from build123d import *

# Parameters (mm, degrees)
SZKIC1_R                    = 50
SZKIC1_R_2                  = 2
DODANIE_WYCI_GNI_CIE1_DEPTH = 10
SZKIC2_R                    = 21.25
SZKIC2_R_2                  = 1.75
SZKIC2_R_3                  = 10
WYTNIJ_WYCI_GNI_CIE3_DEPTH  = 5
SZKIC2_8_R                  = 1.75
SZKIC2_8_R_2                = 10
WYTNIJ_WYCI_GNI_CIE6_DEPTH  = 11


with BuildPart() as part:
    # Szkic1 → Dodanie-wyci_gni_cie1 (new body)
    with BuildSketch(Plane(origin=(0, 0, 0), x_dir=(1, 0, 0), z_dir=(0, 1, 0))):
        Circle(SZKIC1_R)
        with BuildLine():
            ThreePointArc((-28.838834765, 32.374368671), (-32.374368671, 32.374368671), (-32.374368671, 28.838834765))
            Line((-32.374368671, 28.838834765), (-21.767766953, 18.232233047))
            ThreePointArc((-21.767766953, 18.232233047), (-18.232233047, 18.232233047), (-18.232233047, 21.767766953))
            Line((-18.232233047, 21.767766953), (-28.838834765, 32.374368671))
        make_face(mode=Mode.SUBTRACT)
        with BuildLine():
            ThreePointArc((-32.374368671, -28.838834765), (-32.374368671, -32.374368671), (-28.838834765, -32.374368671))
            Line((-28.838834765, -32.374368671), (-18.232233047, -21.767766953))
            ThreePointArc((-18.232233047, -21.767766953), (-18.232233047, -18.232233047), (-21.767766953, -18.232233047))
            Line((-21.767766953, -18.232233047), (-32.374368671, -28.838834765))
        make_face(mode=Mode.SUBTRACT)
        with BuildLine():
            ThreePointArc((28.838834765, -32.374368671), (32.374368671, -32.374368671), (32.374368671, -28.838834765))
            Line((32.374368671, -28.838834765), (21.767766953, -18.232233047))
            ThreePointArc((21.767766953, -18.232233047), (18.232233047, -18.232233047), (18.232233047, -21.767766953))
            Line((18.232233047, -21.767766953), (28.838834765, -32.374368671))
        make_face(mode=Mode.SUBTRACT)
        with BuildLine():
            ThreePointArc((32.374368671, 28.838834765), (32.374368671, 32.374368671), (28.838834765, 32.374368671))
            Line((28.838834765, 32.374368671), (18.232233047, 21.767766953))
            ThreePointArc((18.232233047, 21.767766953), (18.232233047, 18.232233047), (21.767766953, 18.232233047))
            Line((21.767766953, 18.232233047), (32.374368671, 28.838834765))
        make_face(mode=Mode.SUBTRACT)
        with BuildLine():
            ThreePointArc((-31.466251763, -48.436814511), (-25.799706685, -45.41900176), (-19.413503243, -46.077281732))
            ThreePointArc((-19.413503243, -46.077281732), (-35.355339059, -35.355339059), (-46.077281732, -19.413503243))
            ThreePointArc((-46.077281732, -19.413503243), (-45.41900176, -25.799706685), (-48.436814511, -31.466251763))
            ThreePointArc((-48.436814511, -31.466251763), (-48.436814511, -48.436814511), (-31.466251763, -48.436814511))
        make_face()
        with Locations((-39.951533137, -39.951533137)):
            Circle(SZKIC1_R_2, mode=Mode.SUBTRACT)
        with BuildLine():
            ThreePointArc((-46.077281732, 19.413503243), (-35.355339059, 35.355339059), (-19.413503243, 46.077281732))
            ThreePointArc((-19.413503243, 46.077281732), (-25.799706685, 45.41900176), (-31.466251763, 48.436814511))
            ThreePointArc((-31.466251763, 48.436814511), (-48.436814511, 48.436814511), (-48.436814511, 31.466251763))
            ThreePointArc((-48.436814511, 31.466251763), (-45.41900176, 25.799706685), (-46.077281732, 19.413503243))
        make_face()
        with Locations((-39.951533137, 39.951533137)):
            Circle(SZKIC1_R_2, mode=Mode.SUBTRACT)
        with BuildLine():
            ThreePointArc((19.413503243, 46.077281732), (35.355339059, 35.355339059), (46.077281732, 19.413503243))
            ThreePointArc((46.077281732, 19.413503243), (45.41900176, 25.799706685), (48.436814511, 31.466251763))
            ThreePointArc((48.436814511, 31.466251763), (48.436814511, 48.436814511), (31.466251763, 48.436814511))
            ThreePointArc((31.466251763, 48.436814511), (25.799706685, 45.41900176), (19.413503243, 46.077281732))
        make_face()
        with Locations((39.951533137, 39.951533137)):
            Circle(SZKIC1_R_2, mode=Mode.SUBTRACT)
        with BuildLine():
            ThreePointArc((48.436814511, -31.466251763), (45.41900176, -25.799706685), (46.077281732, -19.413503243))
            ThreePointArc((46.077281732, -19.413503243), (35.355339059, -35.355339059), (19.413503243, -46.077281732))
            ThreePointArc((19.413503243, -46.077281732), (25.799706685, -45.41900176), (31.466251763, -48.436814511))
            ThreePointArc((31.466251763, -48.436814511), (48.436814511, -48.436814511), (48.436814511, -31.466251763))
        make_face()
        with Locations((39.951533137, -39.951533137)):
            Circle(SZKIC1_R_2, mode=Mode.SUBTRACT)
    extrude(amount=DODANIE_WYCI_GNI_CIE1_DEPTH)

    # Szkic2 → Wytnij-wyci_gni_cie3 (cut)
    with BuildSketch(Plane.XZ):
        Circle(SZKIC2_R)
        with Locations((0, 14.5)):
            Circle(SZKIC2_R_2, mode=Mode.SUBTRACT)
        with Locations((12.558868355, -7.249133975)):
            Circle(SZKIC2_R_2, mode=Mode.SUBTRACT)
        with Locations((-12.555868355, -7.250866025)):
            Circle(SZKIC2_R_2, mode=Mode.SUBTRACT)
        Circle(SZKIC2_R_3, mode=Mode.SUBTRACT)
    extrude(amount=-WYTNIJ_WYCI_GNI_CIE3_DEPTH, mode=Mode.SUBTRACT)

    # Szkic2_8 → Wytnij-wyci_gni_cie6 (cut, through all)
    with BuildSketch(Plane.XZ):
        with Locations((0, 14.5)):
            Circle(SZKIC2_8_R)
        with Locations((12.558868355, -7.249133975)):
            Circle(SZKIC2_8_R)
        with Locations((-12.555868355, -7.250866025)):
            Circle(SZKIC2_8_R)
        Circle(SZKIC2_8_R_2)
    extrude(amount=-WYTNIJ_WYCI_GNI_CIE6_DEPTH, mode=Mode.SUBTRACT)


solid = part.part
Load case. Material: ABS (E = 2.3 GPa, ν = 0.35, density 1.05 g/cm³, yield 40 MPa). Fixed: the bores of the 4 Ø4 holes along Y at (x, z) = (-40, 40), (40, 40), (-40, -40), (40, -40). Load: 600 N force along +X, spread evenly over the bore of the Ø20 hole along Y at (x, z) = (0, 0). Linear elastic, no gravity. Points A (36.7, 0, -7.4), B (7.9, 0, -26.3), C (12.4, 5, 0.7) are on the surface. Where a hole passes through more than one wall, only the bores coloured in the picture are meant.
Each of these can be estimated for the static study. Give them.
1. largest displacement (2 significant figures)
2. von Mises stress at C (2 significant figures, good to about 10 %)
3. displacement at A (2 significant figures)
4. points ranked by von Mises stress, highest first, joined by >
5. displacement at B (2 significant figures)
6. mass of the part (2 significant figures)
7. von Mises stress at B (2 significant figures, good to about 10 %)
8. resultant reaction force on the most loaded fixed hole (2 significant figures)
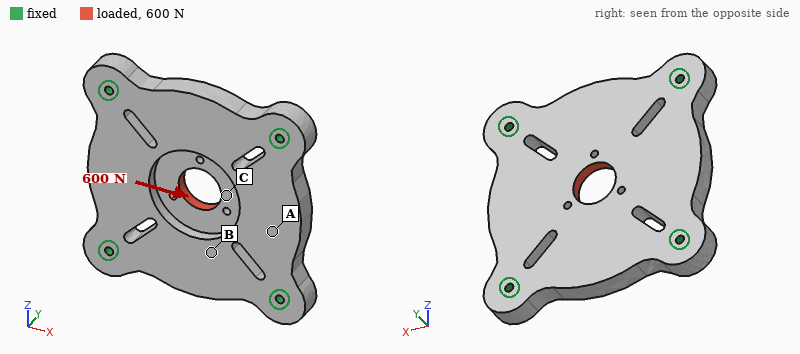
37 µm
1.8 MPa
20 µm
C > B > A
12 µm
86 g
0.79 MPa
170 N
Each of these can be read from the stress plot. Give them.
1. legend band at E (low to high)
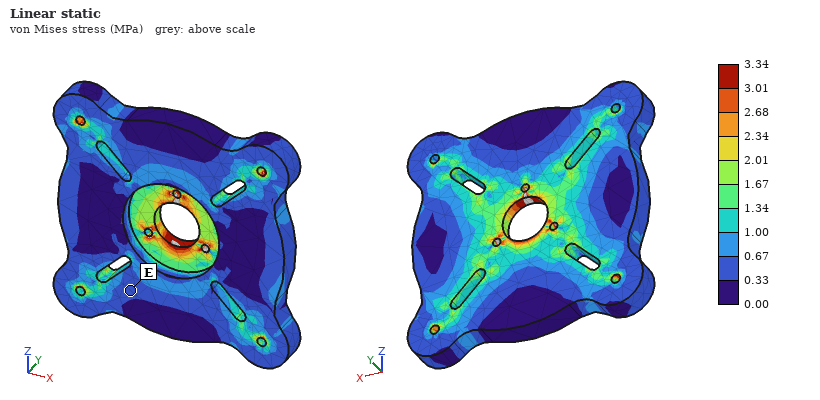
0.33 to 0.67 MPa
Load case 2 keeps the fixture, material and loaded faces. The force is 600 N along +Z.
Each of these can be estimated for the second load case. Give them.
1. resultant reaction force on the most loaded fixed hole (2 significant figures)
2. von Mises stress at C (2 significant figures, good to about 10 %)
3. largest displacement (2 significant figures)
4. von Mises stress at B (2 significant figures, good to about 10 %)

170 N
2.9 MPa
39 µm
0.33 MPa
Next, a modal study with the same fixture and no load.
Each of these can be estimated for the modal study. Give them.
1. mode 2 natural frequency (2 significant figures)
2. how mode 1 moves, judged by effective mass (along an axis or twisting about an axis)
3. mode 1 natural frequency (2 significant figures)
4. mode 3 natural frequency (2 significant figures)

2100 Hz
along Y
1400 Hz
2100 Hz
